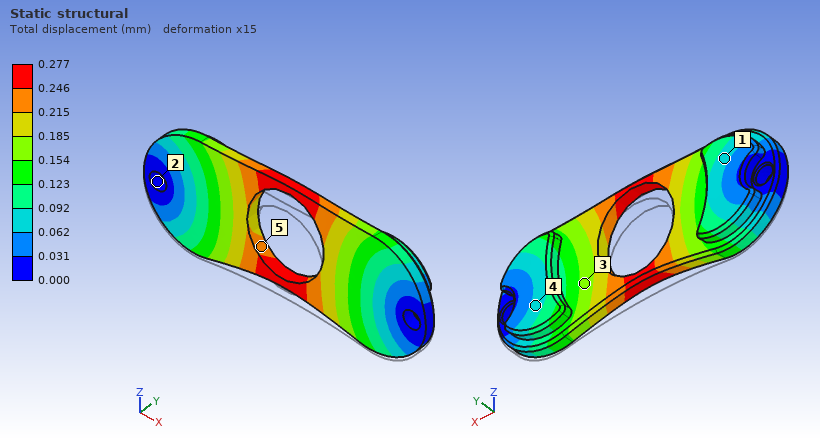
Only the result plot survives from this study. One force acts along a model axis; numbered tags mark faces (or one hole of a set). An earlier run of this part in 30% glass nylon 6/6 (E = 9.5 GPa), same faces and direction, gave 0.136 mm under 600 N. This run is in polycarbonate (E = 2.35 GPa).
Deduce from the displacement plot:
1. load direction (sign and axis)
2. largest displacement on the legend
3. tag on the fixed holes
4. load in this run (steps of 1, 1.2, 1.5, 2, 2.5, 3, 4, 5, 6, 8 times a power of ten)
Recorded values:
+Z
0.277 mm
2
300 N
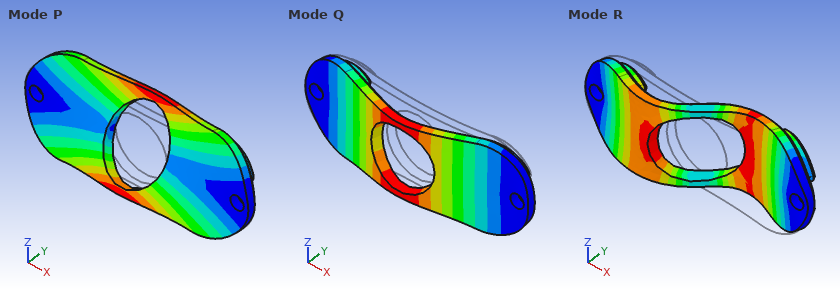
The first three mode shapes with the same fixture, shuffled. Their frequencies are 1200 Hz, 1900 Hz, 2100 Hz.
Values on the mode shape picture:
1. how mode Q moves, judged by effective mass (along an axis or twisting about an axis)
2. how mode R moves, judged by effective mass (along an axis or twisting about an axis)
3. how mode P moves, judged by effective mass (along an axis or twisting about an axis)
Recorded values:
along Y
twisting about Z
twisting about X
